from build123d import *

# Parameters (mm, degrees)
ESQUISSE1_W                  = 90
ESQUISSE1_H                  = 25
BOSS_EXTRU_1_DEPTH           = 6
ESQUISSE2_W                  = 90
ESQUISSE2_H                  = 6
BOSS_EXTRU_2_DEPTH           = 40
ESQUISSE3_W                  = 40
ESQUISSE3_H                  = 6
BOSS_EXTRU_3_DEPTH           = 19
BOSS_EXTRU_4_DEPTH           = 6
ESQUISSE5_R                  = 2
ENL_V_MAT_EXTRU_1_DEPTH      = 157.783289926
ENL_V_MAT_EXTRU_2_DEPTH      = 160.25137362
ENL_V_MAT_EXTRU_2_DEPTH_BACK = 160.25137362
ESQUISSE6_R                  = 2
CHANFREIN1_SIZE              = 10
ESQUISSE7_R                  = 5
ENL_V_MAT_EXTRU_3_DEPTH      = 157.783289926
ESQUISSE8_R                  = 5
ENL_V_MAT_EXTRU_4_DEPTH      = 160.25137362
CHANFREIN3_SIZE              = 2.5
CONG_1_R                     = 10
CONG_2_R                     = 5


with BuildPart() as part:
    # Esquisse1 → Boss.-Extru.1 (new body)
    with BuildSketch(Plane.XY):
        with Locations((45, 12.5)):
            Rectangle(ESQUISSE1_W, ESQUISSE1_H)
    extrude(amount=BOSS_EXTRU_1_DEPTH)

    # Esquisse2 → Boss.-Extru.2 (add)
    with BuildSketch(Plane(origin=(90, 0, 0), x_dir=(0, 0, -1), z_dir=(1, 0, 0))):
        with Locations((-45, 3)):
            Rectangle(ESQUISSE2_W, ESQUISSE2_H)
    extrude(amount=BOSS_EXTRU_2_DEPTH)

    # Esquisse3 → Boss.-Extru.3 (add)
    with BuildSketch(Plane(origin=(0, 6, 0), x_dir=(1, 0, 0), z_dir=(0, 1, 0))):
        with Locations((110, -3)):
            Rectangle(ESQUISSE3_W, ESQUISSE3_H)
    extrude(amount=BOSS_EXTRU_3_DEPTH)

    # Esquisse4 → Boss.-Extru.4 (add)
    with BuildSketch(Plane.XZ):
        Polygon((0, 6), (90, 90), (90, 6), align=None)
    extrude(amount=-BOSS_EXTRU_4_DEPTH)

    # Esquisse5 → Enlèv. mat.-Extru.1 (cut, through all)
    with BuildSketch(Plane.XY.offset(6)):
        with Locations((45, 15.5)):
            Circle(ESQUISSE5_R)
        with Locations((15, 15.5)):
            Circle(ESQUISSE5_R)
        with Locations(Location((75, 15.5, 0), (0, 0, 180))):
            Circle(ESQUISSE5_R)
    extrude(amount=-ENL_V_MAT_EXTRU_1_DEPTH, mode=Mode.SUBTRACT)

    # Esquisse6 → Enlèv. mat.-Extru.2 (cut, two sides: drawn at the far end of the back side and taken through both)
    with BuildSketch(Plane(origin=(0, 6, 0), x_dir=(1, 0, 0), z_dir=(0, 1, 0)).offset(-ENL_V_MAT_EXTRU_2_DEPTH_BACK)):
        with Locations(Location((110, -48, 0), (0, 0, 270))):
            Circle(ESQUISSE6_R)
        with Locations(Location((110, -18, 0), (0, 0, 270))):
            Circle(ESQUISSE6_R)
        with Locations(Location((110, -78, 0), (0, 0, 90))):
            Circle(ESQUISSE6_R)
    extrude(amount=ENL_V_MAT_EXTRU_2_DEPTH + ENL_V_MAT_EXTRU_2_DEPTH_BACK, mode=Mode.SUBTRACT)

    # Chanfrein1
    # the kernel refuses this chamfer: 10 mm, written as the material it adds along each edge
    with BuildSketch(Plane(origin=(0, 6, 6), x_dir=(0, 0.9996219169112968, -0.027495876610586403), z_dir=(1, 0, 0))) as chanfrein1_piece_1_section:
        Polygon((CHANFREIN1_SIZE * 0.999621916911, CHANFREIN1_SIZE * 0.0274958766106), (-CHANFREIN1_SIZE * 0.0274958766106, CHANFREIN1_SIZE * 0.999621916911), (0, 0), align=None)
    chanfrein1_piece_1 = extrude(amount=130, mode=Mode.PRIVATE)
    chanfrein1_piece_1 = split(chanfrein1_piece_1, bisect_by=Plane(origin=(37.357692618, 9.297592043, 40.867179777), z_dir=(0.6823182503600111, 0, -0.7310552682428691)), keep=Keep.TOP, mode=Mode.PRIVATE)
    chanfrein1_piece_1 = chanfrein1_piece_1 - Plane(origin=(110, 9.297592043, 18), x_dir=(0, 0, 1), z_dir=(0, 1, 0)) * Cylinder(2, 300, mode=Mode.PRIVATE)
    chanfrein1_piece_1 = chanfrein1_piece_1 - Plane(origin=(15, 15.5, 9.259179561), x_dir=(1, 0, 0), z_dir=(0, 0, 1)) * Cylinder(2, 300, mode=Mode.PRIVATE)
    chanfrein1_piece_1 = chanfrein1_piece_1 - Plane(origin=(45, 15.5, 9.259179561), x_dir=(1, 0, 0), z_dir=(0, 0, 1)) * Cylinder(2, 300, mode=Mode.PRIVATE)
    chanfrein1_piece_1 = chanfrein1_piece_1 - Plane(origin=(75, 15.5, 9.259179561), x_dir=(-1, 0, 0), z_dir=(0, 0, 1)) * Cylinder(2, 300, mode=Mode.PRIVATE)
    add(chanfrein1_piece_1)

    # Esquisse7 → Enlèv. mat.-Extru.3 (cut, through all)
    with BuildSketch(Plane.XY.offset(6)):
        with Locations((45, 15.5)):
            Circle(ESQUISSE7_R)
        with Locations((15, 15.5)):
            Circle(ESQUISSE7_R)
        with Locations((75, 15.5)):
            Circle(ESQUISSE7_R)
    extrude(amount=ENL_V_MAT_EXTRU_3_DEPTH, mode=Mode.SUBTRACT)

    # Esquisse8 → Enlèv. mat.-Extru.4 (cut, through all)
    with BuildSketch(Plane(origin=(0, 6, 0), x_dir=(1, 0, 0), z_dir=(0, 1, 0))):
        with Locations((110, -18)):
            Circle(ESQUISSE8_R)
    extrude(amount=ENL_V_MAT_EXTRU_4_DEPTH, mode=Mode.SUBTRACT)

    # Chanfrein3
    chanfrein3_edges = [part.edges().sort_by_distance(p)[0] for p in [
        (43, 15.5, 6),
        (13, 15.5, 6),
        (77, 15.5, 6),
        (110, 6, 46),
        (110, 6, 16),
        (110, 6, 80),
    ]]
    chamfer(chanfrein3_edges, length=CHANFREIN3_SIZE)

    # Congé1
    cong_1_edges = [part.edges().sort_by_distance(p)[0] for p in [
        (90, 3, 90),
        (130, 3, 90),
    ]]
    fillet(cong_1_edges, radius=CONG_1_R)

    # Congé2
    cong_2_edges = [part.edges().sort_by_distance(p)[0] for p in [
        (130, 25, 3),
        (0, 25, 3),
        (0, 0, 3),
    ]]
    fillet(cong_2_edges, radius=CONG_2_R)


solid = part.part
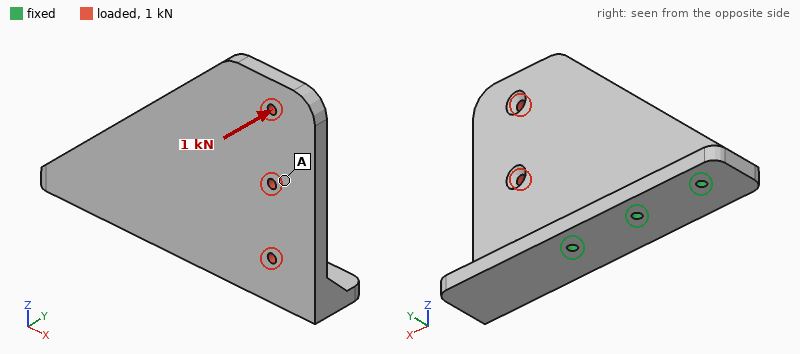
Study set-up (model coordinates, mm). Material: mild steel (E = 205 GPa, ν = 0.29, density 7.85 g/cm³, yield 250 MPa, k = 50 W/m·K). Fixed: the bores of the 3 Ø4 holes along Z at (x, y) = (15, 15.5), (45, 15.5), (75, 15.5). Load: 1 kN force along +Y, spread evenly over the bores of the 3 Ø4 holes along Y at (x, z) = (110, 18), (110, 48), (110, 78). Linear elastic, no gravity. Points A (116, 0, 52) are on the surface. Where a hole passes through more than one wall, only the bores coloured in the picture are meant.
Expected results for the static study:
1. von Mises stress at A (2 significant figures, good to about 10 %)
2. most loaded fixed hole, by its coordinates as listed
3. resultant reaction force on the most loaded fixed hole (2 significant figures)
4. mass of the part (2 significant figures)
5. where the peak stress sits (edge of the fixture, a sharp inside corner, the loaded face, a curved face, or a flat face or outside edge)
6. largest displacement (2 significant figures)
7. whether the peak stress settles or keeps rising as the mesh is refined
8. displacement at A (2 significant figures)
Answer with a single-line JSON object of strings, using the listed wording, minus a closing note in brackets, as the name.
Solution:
{"von Mises stress at A": "28 MPa", "most loaded fixed hole, by its coordinates as listed": "(75, 15.5)", "resultant reaction force on the most loaded fixed hole": "1.9 kN", "mass of the part": "530 g", "where the peak stress sits": "edge of the fixture", "largest displacement": "0.52 mm", "whether the peak stress settles or keeps rising as the mesh is refined": "keeps rising", "displacement at A": "0.27 mm"}
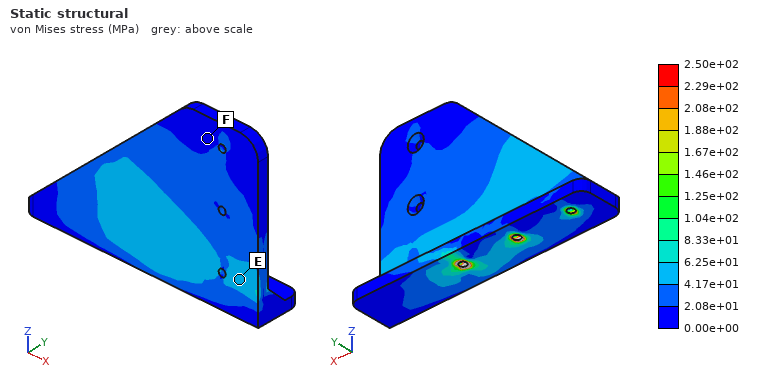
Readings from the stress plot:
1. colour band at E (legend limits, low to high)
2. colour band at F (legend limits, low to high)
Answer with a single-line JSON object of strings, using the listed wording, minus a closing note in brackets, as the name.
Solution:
{"colour band at E": "4.17e+01 to 6.25e+01 MPa", "colour band at F": "0.00e+00 to 2.08e+01 MPa"}
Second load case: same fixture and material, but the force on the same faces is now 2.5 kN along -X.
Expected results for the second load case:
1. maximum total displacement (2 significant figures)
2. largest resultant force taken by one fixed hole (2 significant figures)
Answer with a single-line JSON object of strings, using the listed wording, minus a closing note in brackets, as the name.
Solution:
{"maximum total displacement": "67 µm", "largest resultant force taken by one fixed hole": "2.2 kN"}
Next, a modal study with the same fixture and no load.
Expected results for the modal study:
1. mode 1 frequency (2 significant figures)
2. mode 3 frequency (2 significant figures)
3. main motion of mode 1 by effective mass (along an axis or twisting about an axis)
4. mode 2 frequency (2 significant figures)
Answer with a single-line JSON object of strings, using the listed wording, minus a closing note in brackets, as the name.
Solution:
{"mode 1 frequency": "620 Hz", "mode 3 frequency": "2300 Hz", "main motion of mode 1 by effective mass": "along Y", "mode 2 frequency": "2100 Hz"}
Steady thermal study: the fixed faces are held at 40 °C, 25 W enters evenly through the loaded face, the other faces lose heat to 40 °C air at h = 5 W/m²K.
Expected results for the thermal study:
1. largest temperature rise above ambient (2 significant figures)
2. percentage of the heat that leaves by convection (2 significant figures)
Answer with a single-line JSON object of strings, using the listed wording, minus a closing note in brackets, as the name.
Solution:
{"largest temperature rise above ambient": "79 K", "percentage of the heat that leaves by convection": "15 %"}
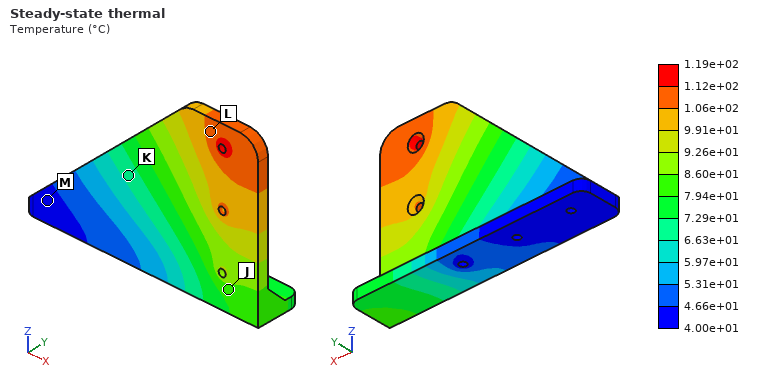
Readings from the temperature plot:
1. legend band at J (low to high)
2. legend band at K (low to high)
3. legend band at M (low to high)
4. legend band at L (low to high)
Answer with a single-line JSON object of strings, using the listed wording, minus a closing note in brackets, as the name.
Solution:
{"legend band at J": "7.94e+01 to 8.60e+01 °C", "legend band at K": "6.63e+01 to 7.29e+01 °C", "legend band at M": "4.00e+01 to 4.66e+01 °C", "legend band at L": "1.06e+02 to 1.12e+02 °C"}
